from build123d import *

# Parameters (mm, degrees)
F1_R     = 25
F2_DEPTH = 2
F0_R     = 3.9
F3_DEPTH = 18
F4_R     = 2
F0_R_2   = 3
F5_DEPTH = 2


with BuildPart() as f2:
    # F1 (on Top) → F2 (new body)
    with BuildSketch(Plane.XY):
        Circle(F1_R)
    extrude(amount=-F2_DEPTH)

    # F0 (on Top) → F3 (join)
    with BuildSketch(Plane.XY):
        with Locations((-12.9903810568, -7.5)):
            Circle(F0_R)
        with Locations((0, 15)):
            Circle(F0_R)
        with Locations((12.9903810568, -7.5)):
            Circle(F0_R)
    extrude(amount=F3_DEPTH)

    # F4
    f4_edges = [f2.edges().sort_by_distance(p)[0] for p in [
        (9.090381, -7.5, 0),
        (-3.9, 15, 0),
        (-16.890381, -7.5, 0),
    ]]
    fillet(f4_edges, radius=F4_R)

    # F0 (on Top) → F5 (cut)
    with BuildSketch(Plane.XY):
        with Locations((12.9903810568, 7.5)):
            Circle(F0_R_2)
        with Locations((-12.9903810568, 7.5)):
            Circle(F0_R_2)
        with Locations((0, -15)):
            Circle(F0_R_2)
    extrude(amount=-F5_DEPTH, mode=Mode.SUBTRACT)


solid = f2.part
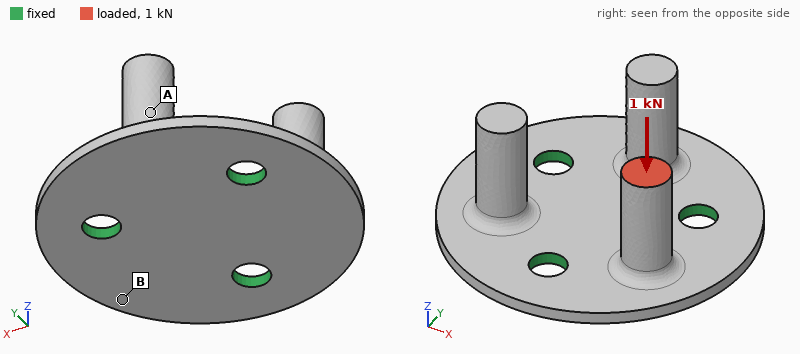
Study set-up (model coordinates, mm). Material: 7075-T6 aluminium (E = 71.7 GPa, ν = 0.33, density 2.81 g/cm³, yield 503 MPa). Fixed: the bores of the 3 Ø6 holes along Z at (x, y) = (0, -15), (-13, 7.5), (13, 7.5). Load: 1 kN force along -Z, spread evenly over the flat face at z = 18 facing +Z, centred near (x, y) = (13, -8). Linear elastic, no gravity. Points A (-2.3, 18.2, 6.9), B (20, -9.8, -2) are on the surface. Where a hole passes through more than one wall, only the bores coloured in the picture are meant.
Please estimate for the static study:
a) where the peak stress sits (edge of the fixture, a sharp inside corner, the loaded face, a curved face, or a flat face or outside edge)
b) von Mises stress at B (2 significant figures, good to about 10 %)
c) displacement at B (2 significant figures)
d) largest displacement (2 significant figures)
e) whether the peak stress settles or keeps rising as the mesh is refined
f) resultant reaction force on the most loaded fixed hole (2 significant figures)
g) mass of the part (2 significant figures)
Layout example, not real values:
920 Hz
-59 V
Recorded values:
edge of the fixture
78 MPa
0.21 mm
0.29 mm
keeps rising
540 N
18 g
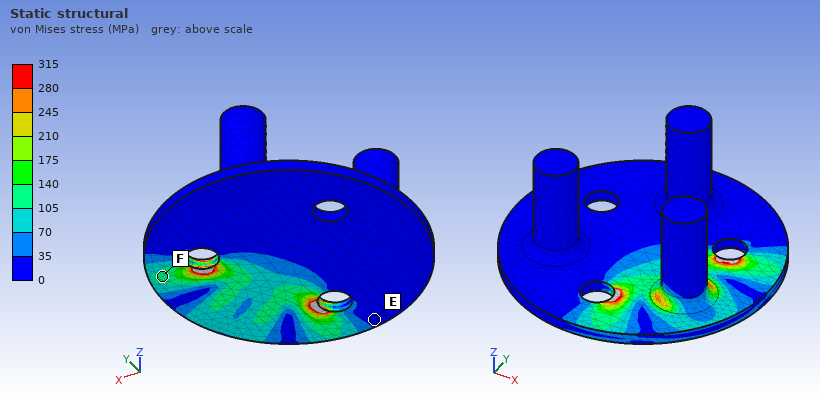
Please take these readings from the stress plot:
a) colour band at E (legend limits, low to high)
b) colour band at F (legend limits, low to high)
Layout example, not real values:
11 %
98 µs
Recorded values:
0 to 35 MPa
105 to 140 MPa
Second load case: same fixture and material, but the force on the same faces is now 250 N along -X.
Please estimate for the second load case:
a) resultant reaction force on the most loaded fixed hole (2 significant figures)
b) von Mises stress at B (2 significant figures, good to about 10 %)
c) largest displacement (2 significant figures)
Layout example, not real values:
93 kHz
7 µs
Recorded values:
170 N
63 MPa
0.30 mm
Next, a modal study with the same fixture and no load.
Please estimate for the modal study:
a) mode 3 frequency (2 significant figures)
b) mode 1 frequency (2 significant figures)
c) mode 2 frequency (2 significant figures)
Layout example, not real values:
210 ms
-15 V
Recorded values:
4200 Hz
4000 Hz
4200 Hz
